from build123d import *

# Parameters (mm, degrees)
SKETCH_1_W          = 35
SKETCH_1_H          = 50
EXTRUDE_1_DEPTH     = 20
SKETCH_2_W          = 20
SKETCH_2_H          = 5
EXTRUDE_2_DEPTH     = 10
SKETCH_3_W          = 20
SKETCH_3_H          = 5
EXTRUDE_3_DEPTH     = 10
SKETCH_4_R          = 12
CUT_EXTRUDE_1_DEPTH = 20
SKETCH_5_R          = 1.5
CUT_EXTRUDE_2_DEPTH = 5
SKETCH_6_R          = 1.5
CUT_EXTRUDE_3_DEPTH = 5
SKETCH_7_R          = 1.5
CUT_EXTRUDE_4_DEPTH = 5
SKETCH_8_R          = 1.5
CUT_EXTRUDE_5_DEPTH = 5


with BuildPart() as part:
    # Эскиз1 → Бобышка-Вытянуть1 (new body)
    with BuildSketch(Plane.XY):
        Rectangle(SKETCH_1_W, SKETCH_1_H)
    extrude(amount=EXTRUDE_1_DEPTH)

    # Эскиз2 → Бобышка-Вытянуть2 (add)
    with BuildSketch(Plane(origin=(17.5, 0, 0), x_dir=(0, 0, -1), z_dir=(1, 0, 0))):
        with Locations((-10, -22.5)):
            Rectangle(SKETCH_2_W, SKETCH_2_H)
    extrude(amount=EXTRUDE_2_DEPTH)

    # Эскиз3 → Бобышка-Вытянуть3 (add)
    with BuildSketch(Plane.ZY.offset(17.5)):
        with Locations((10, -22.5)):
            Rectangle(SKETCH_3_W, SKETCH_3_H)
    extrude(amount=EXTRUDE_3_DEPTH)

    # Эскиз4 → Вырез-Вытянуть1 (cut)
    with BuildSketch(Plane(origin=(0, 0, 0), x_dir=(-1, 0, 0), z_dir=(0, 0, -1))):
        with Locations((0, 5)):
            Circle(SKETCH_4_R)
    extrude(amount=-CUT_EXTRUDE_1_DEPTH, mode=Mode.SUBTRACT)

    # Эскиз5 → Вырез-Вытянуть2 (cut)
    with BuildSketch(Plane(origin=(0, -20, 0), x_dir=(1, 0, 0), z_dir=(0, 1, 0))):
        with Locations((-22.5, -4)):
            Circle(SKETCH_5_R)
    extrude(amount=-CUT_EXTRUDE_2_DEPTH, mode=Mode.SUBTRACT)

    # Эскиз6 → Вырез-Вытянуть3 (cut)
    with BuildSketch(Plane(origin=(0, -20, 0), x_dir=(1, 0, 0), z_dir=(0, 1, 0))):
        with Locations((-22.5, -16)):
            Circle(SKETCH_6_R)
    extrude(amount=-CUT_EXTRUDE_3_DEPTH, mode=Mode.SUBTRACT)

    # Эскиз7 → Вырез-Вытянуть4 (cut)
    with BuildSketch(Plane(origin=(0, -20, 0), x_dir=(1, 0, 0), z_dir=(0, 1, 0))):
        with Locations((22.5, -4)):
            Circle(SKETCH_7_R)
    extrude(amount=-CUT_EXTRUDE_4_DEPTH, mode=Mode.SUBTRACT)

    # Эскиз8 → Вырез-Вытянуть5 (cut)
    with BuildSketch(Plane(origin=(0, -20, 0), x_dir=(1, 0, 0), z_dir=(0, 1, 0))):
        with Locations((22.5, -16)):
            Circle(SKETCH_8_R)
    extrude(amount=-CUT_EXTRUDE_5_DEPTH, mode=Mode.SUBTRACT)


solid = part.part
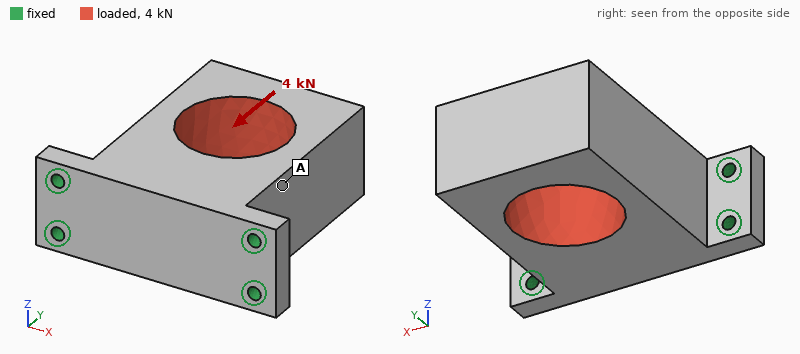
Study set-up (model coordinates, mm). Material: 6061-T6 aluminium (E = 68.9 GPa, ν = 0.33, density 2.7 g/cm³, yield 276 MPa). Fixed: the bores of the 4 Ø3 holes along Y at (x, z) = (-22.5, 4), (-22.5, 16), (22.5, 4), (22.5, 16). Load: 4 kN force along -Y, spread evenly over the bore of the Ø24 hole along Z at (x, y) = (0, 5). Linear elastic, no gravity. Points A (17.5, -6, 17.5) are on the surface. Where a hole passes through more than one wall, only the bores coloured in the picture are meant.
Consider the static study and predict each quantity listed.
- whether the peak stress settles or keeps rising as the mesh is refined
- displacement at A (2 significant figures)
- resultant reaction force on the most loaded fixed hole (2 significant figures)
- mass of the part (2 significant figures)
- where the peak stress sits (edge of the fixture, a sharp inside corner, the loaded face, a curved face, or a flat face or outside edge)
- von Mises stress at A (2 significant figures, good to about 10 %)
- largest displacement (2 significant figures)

keeps rising
13 µm
1.1 kN
75 g
edge of the fixture
14 MPa
19 µm
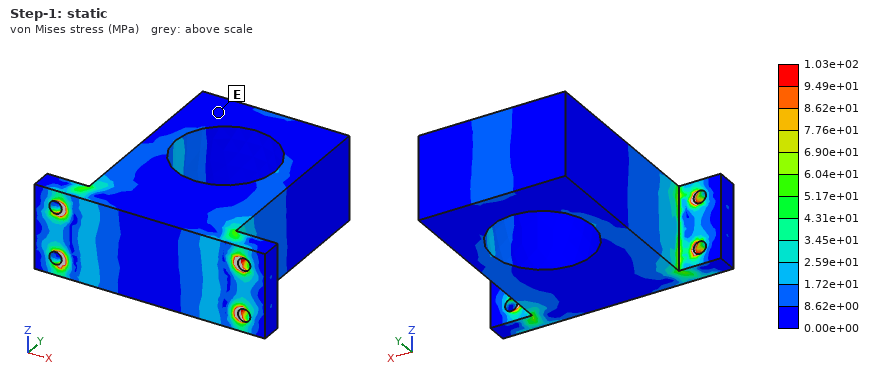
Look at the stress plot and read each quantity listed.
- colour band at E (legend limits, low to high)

0.00e+00 to 8.62e+00 MPa
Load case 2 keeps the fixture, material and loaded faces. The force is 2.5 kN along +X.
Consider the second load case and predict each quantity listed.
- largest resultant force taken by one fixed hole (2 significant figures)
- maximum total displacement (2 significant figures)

1.1 kN
54 µm
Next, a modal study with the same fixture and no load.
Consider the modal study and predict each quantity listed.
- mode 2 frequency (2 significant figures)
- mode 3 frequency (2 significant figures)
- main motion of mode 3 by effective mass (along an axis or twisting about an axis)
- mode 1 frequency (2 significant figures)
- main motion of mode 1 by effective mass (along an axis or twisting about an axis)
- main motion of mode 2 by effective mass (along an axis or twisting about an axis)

5300 Hz
9200 Hz
twisting about Y
2600 Hz
along Z
along X
